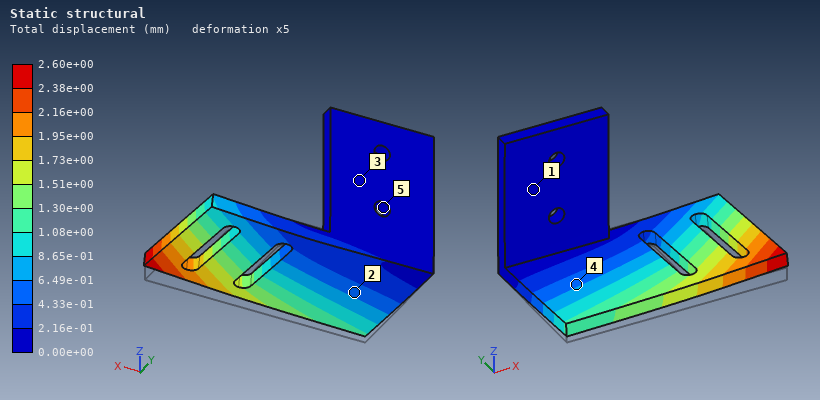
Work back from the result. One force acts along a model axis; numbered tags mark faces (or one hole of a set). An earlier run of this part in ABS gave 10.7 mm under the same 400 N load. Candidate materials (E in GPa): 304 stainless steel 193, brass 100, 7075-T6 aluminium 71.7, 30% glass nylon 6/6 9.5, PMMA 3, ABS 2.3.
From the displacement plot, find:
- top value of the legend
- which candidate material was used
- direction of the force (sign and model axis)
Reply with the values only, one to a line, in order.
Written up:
2.60e+00 mm
30% glass nylon 6/6
+Z
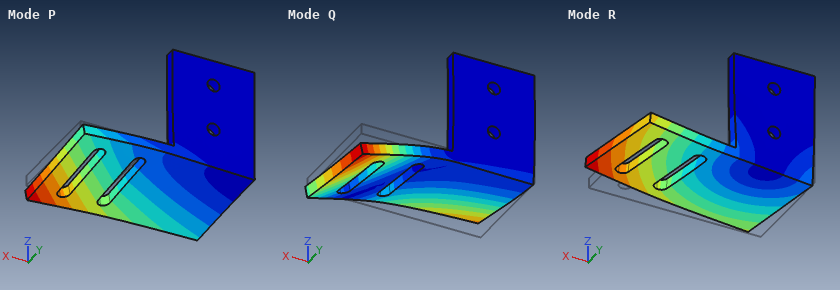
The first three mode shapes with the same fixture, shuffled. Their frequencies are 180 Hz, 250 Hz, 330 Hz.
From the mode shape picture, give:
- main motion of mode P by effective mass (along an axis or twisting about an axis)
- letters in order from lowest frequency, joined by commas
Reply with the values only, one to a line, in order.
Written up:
along Z
P, R, Q
